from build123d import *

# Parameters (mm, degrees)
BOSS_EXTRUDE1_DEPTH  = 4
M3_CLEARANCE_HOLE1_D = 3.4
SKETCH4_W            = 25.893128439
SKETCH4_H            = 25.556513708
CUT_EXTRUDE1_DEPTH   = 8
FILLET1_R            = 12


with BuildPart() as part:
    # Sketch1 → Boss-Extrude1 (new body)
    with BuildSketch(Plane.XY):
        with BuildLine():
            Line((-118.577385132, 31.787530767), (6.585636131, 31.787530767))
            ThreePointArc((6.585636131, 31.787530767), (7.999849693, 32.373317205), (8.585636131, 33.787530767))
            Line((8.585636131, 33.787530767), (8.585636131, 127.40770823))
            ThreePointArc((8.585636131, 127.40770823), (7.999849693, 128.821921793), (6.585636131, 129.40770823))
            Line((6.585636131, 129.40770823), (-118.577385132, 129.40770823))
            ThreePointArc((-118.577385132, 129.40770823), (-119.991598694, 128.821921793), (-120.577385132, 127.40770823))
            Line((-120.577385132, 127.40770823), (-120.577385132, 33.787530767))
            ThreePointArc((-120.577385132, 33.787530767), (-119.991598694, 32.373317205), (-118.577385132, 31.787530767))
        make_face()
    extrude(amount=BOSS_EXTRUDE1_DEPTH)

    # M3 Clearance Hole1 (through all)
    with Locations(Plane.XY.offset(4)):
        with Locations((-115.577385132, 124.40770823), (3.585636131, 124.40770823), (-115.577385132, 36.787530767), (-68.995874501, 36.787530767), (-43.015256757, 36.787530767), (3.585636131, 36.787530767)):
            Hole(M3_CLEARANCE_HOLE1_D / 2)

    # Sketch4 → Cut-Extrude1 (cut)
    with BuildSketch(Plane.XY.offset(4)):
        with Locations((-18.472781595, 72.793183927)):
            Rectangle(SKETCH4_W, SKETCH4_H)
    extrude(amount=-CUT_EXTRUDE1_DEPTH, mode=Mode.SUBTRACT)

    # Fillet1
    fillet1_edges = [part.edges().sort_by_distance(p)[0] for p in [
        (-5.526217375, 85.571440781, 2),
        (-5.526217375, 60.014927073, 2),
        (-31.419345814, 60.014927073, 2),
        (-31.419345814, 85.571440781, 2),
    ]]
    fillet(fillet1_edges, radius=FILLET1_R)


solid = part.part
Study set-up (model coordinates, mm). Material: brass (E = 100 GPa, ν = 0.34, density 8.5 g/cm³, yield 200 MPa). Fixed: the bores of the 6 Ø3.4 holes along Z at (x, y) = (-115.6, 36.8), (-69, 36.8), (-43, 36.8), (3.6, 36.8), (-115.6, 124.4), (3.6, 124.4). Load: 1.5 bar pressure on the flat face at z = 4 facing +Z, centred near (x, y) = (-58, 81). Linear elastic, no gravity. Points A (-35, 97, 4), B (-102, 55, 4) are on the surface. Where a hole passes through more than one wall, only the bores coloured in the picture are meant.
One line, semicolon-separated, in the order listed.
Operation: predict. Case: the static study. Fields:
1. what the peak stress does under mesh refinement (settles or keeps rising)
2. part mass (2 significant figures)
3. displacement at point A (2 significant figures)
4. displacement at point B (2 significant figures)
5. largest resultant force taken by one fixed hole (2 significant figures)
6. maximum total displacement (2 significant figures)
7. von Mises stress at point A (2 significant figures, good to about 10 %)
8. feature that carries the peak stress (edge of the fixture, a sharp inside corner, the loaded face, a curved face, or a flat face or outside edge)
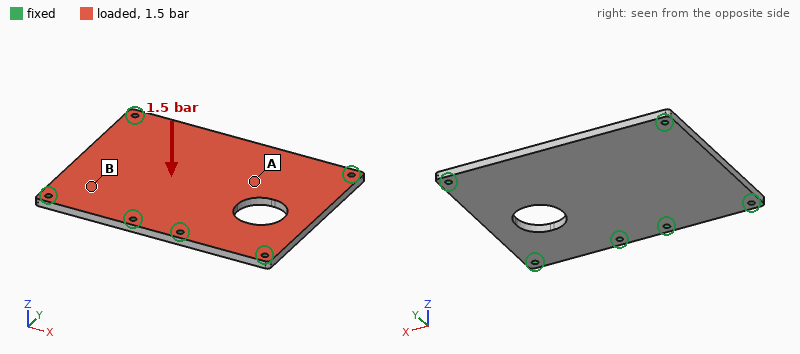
keeps rising; 410 g; 0.15 mm; 0.041 mm; 420 N; 0.20 mm; 28 MPa; edge of the fixture
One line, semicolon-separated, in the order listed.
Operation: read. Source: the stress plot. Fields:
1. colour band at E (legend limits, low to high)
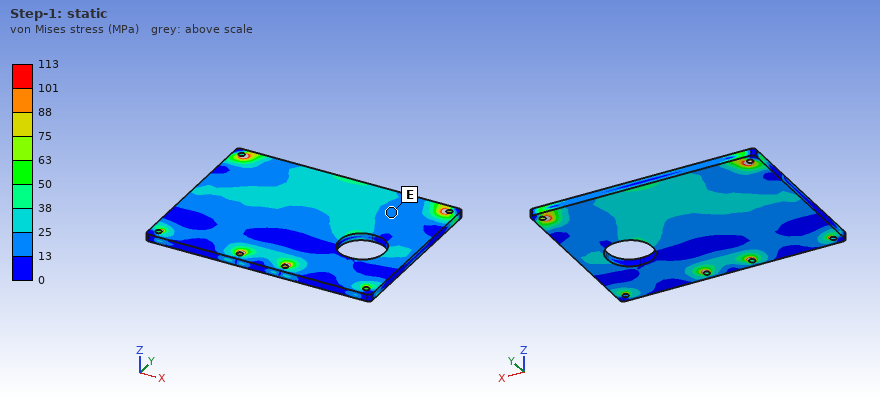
13 to 25 MPa
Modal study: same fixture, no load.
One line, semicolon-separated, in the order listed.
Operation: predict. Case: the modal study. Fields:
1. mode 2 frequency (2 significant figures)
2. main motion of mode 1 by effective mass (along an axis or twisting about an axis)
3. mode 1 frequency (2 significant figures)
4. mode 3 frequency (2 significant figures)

1700 Hz; along Z; 940 Hz; 1700 Hz
